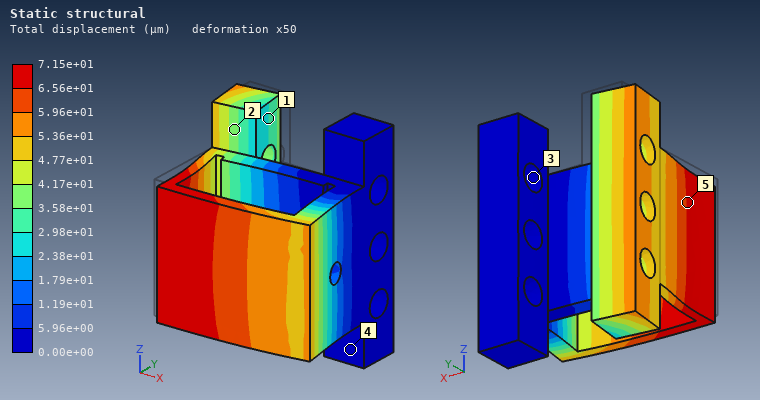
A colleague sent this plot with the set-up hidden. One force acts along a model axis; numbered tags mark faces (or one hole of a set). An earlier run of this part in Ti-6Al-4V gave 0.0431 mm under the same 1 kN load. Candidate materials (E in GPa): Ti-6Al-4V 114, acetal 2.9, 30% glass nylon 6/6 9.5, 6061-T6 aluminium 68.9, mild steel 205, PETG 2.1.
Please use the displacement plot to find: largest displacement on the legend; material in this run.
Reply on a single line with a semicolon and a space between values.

7.15e+01 µm; 6061-T6 aluminium
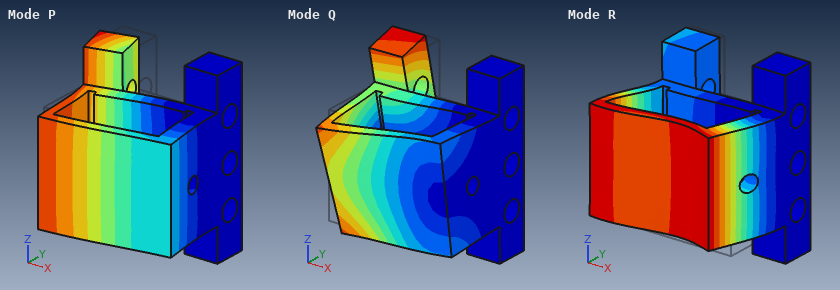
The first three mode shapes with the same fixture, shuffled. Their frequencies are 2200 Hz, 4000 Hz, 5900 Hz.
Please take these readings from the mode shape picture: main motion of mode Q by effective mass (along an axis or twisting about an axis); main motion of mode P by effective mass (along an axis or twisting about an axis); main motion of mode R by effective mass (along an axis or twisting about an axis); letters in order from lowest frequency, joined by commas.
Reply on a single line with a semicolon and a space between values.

twisting about X; along Y; along X; P, Q, R
